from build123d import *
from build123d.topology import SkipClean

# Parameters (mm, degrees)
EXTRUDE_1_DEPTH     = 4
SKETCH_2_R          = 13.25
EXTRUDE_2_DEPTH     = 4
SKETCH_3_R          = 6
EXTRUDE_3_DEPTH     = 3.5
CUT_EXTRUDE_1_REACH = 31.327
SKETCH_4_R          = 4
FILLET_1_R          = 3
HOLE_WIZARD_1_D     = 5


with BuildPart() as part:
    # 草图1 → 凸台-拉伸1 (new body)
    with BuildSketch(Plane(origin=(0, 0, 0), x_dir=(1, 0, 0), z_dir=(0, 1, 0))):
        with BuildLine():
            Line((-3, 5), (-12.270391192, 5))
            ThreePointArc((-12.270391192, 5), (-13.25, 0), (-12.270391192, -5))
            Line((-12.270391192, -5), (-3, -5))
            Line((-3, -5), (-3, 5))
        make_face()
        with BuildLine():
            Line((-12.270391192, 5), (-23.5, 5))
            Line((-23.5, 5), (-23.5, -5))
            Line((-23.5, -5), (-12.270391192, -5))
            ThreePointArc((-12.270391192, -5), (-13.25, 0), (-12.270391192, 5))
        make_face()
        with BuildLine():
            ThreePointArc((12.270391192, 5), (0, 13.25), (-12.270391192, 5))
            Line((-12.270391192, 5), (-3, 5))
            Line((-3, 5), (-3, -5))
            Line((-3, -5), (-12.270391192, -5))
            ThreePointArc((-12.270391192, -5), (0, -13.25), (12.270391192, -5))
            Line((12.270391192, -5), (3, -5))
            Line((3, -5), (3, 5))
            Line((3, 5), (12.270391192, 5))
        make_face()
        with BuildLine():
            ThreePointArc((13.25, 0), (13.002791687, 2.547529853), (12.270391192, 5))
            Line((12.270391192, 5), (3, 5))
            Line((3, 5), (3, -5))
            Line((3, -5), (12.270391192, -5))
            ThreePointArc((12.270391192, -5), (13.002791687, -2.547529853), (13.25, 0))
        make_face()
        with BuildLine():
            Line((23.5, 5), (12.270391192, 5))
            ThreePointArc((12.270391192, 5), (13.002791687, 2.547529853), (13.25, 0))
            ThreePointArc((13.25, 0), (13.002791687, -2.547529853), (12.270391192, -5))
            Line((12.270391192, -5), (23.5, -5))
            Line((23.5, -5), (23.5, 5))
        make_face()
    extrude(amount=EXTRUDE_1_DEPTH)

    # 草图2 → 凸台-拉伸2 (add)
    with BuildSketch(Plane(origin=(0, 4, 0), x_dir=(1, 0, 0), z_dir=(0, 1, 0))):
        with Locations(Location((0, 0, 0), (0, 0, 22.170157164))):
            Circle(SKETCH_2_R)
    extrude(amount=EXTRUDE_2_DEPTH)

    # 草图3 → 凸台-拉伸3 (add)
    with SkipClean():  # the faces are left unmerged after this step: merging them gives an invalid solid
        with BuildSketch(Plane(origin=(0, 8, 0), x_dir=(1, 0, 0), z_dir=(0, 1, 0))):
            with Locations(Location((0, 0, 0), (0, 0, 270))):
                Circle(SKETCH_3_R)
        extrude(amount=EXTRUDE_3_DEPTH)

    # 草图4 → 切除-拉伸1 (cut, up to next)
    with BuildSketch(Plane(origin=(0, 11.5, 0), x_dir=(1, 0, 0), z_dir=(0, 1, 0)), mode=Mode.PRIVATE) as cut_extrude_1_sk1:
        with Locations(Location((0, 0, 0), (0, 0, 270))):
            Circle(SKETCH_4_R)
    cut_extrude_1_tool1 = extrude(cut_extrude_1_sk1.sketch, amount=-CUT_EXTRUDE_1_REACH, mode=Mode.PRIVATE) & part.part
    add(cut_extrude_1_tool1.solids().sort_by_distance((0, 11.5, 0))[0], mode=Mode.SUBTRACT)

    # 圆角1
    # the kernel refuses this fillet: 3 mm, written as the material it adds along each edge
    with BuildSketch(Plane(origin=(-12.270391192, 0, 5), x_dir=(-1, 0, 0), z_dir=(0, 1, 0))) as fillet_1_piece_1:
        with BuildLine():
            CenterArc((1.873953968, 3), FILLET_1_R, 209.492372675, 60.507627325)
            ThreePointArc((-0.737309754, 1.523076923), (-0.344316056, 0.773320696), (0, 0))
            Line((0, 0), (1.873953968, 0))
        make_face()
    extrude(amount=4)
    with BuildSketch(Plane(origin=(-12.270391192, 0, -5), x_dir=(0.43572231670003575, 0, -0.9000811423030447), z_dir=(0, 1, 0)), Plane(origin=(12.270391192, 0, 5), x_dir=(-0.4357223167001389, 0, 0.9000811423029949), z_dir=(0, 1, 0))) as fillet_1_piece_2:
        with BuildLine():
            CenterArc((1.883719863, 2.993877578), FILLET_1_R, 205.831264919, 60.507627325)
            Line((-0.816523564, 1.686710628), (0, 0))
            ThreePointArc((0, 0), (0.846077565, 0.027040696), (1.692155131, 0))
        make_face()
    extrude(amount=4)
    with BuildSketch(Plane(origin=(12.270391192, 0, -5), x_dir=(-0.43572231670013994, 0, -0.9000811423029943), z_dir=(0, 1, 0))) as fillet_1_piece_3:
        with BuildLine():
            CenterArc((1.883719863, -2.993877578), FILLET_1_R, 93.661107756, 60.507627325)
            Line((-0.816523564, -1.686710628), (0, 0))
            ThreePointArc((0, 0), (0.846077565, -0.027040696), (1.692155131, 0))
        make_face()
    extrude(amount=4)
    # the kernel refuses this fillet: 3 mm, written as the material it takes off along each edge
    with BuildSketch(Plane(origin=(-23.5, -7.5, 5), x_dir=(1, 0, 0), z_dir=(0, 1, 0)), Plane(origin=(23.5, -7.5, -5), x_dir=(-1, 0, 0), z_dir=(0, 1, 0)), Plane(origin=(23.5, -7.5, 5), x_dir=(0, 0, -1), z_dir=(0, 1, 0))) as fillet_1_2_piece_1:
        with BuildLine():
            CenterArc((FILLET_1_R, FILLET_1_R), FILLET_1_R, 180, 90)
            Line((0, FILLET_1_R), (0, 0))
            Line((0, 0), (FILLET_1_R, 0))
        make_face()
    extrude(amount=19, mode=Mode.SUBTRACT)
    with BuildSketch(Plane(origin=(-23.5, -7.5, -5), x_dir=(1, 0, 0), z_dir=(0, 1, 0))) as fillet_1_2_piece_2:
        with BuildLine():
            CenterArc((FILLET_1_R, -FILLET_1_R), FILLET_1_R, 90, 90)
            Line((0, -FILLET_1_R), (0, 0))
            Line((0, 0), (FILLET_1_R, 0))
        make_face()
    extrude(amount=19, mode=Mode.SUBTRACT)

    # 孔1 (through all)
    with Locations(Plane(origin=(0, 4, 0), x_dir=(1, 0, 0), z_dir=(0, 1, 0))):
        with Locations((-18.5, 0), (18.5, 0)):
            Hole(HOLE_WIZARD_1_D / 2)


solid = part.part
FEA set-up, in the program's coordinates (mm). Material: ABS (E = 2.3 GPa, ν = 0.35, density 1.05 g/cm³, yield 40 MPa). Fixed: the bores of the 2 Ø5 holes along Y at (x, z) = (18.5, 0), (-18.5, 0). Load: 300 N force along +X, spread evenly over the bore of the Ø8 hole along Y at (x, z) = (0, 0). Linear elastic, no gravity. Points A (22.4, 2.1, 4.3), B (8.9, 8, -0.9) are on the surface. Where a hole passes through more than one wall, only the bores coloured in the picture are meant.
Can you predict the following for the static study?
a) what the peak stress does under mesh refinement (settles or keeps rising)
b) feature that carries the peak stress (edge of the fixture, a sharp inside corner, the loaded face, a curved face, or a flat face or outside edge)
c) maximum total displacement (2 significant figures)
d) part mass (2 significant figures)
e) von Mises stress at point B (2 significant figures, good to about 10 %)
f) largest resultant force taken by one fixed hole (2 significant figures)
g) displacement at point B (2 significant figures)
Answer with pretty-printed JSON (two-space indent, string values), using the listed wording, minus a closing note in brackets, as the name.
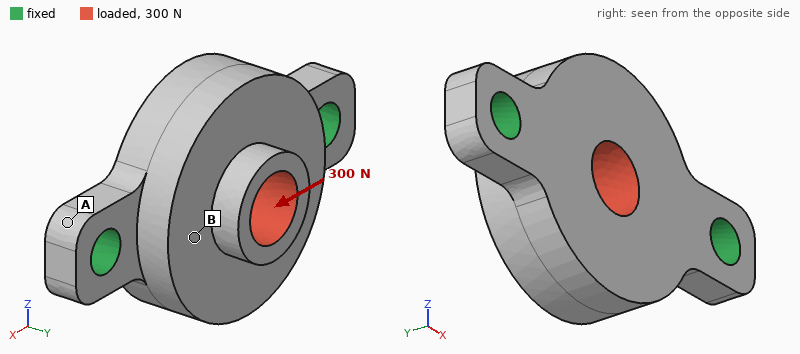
{
  "what the peak stress does under mesh refinement": "keeps rising",
  "feature that carries the peak stress": "edge of the fixture",
  "maximum total displacement": "33 µm",
  "part mass": "5.1 g",
  "von Mises stress at point B": "1.6 MPa",
  "largest resultant force taken by one fixed hole": "150 N",
  "displacement at point B": "17 µm"
}
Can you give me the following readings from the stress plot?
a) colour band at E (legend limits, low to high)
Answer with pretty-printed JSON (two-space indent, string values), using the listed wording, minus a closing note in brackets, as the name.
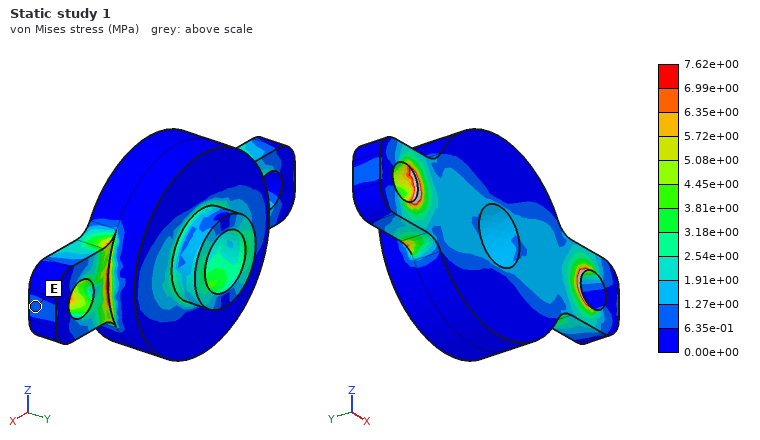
{
  "colour band at E": "6.35e-01 to 1.27e+00 MPa"
}
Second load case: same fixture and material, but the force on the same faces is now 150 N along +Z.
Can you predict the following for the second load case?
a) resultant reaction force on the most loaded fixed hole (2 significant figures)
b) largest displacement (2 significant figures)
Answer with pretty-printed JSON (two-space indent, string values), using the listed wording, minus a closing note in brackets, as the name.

{
  "resultant reaction force on the most loaded fixed hole": "75 N",
  "largest displacement": "0.14 mm"
}
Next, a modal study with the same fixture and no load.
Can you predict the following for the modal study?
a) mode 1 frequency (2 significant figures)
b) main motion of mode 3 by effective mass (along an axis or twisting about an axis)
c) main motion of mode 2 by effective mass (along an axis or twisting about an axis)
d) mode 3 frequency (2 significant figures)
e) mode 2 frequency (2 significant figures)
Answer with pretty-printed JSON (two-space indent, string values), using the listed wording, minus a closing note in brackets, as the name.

{
  "mode 1 frequency": "2500 Hz",
  "main motion of mode 3 by effective mass": "along Z",
  "main motion of mode 2 by effective mass": "along Y",
  "mode 3 frequency": "6900 Hz",
  "mode 2 frequency": "4300 Hz"
}
